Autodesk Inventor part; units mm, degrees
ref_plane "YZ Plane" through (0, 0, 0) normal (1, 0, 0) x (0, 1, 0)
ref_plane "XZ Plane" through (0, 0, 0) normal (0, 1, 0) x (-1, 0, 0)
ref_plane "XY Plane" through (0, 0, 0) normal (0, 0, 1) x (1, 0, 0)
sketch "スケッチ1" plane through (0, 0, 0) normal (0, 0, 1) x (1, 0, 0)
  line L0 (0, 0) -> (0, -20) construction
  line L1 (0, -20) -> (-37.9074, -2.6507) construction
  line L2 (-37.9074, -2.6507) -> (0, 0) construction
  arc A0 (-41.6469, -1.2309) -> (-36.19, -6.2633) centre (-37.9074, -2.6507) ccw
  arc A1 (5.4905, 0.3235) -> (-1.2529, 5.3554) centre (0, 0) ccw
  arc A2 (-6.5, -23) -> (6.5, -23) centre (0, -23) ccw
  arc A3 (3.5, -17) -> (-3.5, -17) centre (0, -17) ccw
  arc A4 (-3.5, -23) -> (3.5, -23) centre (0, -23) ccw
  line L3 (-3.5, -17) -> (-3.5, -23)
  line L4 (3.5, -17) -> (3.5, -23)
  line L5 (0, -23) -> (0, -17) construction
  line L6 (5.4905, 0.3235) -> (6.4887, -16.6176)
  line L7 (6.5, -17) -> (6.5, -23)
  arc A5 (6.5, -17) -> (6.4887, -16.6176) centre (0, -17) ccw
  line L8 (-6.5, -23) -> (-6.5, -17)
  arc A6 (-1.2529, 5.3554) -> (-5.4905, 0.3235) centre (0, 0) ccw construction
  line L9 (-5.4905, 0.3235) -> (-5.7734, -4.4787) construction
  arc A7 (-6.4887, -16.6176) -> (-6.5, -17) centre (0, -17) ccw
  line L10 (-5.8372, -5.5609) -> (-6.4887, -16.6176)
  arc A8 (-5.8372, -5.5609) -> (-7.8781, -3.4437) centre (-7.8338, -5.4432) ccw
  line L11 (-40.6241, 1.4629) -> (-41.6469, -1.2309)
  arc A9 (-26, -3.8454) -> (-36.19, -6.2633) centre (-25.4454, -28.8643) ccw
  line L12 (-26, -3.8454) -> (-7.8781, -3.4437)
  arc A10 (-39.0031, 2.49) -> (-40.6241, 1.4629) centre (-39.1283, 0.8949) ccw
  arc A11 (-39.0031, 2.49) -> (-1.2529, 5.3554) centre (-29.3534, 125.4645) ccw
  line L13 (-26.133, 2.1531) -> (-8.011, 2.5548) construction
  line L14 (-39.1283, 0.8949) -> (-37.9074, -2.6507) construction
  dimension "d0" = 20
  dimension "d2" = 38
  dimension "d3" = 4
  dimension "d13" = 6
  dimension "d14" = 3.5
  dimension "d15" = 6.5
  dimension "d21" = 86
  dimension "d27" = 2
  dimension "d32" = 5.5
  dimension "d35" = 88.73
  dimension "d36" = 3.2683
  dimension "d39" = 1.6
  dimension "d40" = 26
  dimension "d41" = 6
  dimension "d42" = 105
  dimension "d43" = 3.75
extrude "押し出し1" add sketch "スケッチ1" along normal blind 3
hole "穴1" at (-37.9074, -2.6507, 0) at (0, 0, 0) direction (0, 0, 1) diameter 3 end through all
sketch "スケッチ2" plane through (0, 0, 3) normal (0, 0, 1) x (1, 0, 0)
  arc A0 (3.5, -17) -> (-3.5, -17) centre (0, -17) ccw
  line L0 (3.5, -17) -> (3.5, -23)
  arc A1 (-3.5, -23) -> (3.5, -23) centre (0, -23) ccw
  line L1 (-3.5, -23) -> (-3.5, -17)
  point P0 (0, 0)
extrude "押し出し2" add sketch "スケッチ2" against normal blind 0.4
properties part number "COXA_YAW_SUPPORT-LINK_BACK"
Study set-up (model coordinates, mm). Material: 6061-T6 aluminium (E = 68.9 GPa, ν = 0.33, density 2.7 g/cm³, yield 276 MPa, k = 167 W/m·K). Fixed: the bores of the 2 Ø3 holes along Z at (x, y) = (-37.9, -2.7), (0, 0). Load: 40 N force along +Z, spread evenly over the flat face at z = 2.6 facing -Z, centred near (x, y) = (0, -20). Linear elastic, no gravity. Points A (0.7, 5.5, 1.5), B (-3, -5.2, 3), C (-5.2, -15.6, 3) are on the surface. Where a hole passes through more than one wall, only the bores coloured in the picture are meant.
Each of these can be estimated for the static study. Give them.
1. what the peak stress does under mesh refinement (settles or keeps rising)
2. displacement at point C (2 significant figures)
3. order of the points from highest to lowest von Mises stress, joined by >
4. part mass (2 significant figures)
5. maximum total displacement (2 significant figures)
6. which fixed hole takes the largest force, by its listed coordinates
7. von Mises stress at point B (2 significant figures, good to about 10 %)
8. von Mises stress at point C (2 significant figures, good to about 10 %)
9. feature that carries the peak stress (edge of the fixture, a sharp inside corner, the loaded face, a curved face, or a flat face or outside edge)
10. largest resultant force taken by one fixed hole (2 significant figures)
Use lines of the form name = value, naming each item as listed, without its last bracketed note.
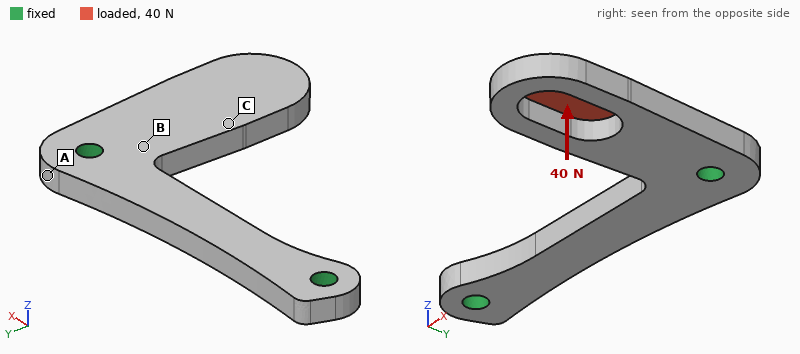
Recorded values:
what the peak stress does under mesh refinement = keeps rising
displacement at point C = 0.037 mm
order of the points from highest to lowest von Mises stress, joined by > = B > C > A
part mass = 4.6 g
maximum total displacement = 0.10 mm
which fixed hole takes the largest force, by its listed coordinates = (0, 0)
von Mises stress at point B = 31 MPa
von Mises stress at point C = 15 MPa
feature that carries the peak stress = edge of the fixture
largest resultant force taken by one fixed hole = 41 N
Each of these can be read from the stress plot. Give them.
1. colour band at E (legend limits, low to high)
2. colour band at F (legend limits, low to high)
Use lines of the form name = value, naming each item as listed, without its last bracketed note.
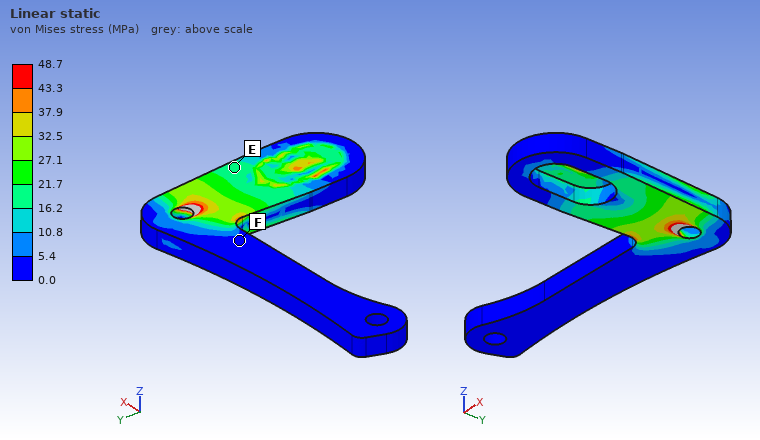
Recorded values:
colour band at E = 16.2 to 21.7 MPa
colour band at F = 0.0 to 5.4 MPa
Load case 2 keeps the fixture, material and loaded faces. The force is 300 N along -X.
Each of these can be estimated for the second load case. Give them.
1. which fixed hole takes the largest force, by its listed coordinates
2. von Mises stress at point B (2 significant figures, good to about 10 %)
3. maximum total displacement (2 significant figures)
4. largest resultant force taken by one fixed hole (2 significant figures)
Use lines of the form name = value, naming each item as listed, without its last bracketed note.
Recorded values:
which fixed hole takes the largest force, by its listed coordinates = (0, 0)
von Mises stress at point B = 39 MPa
maximum total displacement = 0.11 mm
largest resultant force taken by one fixed hole = 310 N
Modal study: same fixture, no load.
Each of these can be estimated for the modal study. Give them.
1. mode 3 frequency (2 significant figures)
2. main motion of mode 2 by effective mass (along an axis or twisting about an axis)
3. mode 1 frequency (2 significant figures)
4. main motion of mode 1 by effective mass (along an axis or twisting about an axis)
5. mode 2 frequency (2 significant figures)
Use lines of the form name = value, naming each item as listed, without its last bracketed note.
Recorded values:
mode 3 frequency = 11 kHz
main motion of mode 2 by effective mass = along X
mode 1 frequency = 3500 Hz
main motion of mode 1 by effective mass = along Z
mode 2 frequency = 8400 Hz
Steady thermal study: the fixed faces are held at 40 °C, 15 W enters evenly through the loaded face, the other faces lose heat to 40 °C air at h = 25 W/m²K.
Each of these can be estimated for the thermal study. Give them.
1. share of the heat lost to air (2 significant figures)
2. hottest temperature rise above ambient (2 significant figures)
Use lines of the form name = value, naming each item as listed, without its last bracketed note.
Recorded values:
share of the heat lost to air = 5.7 %
hottest temperature rise above ambient = 70 K
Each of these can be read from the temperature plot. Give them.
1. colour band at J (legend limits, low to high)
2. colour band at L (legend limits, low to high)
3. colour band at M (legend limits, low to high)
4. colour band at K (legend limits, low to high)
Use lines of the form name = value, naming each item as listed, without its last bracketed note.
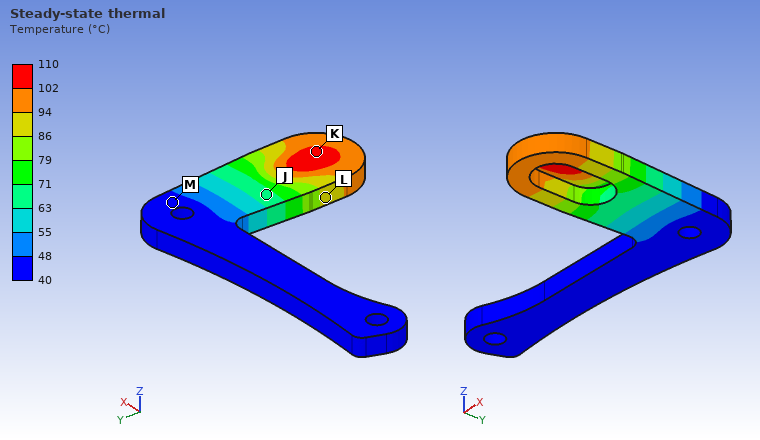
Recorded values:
colour band at J = 63 to 71 °C
colour band at L = 86 to 94 °C
colour band at M = 40 to 48 °C
colour band at K = 102 to 110 °C
